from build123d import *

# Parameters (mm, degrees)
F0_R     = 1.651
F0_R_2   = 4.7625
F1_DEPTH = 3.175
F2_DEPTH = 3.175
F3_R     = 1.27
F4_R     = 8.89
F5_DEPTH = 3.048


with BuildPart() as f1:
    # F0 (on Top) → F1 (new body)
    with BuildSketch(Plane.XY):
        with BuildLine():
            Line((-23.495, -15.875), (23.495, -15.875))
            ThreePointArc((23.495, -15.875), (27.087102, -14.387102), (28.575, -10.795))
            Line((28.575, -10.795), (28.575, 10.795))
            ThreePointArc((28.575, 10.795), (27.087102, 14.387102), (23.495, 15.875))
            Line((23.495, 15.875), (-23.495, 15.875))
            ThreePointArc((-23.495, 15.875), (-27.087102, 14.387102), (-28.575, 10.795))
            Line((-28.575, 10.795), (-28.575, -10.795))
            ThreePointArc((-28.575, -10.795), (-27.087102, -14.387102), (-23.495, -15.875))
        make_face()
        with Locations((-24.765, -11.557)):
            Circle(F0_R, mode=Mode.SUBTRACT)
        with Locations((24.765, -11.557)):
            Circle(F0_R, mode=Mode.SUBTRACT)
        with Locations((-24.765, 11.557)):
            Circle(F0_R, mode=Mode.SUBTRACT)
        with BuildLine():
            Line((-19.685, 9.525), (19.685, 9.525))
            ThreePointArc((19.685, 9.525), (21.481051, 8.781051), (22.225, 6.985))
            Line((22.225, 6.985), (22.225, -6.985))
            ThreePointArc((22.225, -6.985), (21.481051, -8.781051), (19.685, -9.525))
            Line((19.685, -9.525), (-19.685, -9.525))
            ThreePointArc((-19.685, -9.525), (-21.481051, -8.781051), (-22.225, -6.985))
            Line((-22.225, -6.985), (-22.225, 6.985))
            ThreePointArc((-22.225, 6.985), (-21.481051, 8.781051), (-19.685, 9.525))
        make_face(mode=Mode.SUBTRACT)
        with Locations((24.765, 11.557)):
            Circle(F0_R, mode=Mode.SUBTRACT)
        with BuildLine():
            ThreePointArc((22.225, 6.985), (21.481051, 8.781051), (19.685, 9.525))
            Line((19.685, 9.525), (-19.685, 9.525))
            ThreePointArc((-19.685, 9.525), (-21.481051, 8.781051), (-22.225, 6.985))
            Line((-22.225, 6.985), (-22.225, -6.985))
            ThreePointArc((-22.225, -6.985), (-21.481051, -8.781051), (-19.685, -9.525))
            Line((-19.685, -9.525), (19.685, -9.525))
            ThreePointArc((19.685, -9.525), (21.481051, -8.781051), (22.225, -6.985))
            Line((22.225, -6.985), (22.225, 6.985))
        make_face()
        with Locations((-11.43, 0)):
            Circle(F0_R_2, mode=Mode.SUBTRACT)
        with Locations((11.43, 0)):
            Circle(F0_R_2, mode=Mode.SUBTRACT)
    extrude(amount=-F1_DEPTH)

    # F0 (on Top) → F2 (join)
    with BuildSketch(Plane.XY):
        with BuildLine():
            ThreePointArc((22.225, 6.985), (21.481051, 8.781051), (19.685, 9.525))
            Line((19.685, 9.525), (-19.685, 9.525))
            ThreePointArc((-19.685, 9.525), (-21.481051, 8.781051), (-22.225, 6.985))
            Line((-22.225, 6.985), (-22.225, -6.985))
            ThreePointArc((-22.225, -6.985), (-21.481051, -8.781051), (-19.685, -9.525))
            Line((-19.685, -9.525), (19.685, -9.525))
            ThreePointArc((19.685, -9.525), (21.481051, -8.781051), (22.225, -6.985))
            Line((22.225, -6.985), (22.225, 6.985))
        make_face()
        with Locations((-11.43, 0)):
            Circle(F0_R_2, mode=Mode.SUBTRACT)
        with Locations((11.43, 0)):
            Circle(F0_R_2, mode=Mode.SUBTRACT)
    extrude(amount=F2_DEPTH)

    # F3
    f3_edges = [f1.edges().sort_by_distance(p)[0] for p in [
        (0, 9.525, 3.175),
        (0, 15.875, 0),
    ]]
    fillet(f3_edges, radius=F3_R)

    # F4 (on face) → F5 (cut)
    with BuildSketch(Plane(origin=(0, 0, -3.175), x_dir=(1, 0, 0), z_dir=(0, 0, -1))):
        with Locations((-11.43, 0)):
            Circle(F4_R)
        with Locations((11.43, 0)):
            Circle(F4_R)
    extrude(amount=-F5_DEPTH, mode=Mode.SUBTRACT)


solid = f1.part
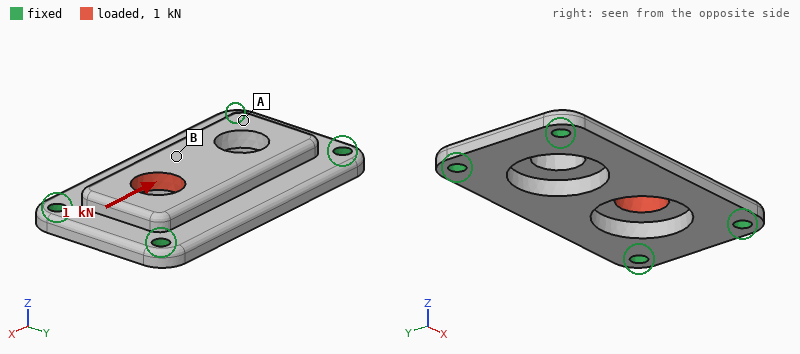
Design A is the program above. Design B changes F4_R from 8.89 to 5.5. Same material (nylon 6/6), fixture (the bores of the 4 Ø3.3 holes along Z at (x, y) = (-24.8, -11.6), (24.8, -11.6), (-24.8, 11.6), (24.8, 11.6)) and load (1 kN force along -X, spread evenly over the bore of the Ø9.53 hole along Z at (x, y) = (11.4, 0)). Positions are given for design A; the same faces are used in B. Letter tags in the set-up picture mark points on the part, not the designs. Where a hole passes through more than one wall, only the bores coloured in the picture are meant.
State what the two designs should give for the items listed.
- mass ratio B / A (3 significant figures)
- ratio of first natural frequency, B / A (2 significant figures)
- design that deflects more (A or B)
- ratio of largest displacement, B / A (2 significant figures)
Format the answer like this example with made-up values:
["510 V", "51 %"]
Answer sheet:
["1.15", "0.99", "A", "0.82"]
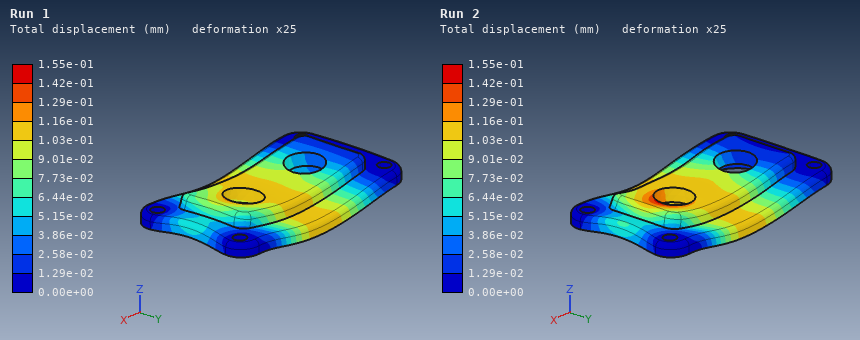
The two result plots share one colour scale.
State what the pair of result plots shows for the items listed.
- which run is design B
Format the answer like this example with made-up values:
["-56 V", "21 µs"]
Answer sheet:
["Run 1"]
